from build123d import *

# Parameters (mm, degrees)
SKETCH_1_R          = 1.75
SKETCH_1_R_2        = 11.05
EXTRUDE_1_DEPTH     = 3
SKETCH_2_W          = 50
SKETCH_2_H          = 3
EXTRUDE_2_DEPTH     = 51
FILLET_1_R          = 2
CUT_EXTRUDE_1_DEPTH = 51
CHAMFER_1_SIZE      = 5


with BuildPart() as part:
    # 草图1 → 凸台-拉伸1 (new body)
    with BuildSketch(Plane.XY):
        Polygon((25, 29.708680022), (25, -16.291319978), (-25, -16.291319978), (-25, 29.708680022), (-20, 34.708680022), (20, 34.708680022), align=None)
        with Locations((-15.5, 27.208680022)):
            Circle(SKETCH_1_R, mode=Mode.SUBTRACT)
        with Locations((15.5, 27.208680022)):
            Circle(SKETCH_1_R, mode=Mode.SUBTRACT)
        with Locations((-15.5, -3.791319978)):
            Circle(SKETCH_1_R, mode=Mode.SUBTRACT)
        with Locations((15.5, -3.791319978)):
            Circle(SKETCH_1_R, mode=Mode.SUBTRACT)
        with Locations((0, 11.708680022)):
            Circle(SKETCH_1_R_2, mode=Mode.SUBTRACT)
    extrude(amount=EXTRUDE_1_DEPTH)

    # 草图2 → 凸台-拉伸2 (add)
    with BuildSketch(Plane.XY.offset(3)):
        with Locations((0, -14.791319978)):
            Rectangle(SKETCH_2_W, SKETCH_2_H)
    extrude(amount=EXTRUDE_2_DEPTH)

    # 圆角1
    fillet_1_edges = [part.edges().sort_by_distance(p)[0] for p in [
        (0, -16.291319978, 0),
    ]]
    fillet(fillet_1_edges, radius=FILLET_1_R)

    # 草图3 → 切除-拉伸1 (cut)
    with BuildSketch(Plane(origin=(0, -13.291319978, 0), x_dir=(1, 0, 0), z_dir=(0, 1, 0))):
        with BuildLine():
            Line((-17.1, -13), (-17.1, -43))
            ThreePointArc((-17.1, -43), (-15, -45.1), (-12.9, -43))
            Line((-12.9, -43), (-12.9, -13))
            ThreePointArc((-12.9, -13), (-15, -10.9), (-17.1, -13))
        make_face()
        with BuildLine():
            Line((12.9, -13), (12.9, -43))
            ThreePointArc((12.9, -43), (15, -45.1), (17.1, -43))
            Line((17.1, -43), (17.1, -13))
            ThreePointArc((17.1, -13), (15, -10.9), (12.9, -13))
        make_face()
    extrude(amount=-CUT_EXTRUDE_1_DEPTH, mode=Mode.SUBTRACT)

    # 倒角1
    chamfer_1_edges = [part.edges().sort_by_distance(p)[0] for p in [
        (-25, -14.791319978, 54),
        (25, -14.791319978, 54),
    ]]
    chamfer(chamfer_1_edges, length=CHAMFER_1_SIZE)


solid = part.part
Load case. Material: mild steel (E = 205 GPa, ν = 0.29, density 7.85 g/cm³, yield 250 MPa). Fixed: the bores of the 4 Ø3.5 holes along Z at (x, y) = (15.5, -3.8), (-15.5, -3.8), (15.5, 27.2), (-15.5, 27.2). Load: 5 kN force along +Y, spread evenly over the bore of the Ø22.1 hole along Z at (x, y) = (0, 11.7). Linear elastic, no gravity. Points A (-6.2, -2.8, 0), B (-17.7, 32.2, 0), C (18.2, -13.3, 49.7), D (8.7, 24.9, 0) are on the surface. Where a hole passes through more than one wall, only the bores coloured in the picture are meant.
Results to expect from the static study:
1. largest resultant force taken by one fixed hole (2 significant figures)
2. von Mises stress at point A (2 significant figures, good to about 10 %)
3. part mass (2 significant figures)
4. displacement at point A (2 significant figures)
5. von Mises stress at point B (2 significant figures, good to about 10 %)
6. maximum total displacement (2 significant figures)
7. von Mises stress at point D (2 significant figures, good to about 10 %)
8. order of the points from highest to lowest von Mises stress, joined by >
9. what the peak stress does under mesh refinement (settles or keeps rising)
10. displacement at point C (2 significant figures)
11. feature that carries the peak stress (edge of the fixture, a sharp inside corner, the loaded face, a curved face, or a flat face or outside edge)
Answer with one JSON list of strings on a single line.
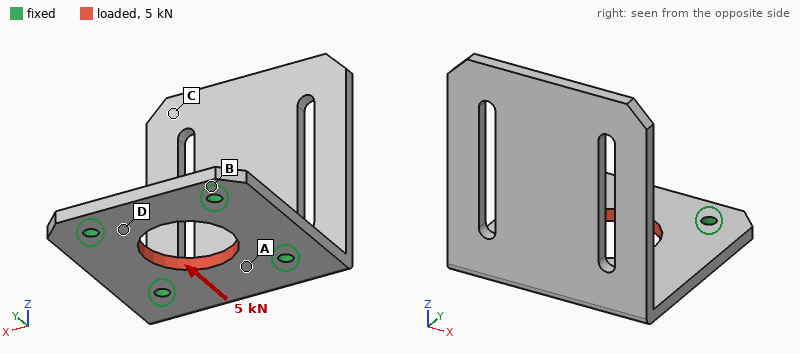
["1.3 kN", "21 MPa", "100 g", "2.1 µm", "14 MPa", "4.3 µm", "30 MPa", "D > A > B > C", "keeps rising", "1.8 µm", "edge of the fixture"]
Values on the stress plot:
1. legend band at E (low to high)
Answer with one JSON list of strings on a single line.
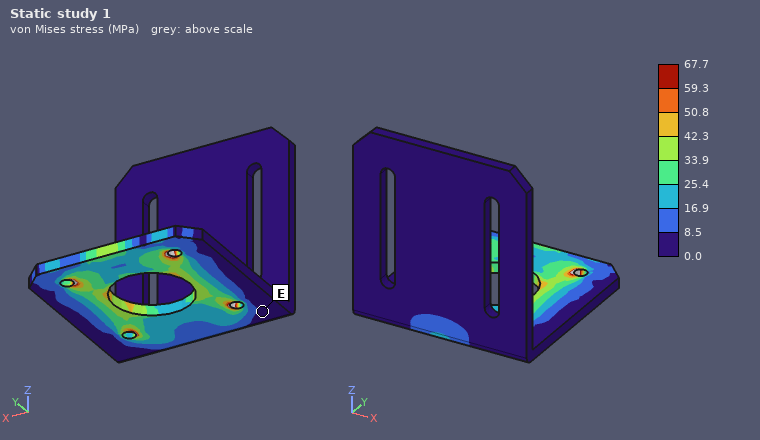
["0.0 to 8.5 MPa"]
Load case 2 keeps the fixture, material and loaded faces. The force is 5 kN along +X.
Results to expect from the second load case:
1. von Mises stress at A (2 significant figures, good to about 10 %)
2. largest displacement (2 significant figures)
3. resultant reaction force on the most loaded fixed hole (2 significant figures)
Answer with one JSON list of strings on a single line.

["29 MPa", "3.8 µm", "1.3 kN"]
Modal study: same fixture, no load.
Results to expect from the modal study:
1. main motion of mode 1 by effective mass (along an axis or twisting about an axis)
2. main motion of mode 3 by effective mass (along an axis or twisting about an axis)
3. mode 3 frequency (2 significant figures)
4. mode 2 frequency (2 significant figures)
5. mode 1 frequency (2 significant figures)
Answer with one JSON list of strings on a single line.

["along Y", "along X", "2800 Hz", "1900 Hz", "690 Hz"]
